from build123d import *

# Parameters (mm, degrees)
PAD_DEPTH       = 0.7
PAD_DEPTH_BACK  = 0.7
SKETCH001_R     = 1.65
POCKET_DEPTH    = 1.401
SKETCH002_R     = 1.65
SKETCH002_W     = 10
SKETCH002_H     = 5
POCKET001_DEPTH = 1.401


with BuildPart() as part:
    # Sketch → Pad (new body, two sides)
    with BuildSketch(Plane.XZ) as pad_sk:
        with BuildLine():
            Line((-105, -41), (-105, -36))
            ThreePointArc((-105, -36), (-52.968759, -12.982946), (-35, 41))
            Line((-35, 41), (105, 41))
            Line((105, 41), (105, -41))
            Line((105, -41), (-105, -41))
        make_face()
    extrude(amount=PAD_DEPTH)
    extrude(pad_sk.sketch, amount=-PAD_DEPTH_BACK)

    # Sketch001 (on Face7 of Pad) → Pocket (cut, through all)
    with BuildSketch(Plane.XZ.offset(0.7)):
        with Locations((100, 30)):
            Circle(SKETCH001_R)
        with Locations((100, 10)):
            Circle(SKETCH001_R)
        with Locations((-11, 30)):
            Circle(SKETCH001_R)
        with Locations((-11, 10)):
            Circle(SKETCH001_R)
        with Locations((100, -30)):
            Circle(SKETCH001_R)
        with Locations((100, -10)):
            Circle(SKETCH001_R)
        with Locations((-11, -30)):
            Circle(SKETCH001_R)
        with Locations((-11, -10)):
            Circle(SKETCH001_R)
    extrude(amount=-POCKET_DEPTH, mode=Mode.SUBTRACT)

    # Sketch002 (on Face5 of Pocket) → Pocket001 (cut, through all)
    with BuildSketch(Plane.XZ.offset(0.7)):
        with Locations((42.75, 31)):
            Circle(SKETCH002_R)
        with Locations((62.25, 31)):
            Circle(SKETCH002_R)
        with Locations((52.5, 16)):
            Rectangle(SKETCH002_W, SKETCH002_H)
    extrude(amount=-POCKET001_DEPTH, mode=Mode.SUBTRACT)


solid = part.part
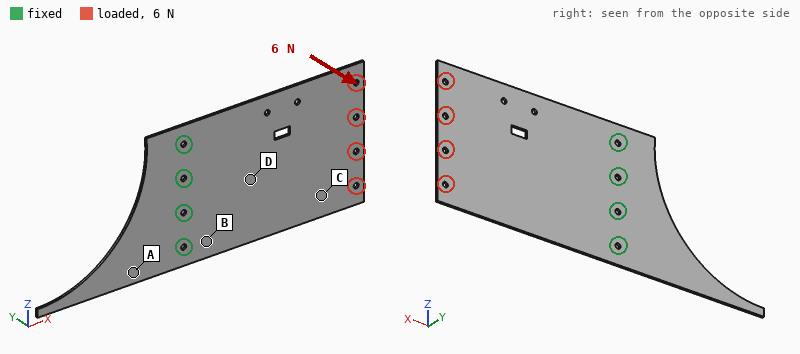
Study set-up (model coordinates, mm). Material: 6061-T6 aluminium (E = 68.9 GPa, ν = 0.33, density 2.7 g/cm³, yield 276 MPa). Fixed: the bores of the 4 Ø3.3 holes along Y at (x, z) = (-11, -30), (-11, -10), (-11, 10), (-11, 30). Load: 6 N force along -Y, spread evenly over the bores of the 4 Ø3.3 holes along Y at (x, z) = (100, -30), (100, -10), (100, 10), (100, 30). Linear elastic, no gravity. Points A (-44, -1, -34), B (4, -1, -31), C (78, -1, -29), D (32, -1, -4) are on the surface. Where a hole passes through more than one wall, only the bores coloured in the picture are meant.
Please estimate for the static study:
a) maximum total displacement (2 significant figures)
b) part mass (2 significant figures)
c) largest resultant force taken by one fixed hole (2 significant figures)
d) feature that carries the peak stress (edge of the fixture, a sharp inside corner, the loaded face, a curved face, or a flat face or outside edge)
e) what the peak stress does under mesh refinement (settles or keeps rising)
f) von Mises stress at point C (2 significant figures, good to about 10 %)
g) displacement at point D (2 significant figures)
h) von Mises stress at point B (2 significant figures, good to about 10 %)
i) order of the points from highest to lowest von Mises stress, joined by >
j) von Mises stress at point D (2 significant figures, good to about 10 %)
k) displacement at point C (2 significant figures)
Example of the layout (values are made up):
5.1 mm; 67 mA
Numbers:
2.2 mm; 48 g; 4.0 N; edge of the fixture; keeps rising; 5.3 MPa; 0.40 mm; 20 MPa; B > D > C > A; 14 MPa; 1.4 mm
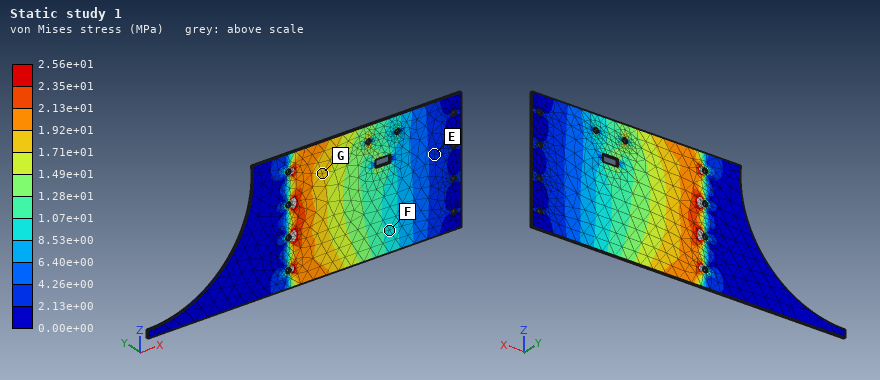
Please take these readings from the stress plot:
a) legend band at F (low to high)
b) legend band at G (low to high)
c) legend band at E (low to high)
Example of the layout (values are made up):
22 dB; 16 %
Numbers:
8.53e+00 to 1.07e+01 MPa; 1.71e+01 to 1.92e+01 MPa; 2.13e+00 to 4.26e+00 MPa
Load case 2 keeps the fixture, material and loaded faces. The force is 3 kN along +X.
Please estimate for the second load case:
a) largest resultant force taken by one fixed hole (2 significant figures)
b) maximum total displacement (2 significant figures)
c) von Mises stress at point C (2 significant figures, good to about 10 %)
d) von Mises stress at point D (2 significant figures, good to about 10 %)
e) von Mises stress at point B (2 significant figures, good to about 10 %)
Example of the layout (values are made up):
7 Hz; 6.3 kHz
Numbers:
810 N; 51 µm; 26 MPa; 28 MPa; 28 MPa
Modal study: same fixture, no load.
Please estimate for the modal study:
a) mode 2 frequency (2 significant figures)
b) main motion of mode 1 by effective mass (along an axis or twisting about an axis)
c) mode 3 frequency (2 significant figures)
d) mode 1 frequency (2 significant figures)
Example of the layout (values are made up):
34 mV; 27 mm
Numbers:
270 Hz; along Y; 280 Hz; 88 Hz
